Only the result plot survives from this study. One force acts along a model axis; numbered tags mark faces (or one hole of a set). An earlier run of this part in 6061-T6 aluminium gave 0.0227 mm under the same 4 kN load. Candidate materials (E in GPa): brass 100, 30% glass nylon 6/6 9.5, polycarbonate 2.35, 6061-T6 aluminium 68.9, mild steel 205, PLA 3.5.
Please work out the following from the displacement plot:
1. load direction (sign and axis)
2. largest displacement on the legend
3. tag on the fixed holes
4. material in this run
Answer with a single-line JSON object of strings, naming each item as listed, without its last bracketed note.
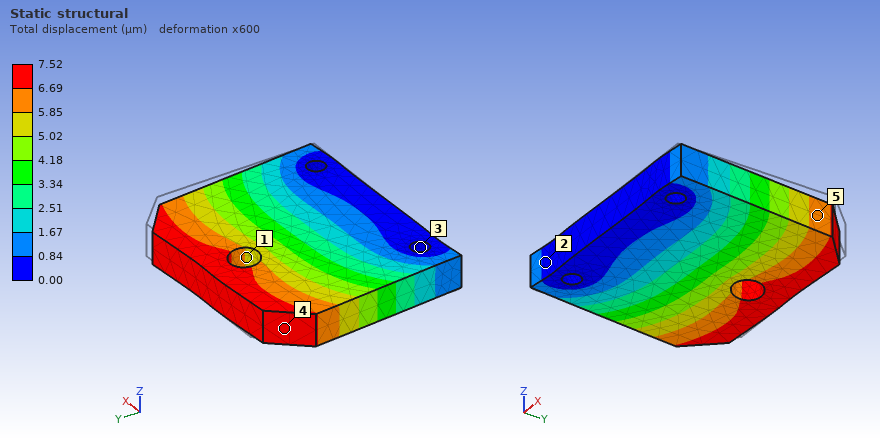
{"load direction": "-X", "largest displacement on the legend": "7.52 µm", "tag on the fixed holes": "3", "material in this run": "mild steel"}
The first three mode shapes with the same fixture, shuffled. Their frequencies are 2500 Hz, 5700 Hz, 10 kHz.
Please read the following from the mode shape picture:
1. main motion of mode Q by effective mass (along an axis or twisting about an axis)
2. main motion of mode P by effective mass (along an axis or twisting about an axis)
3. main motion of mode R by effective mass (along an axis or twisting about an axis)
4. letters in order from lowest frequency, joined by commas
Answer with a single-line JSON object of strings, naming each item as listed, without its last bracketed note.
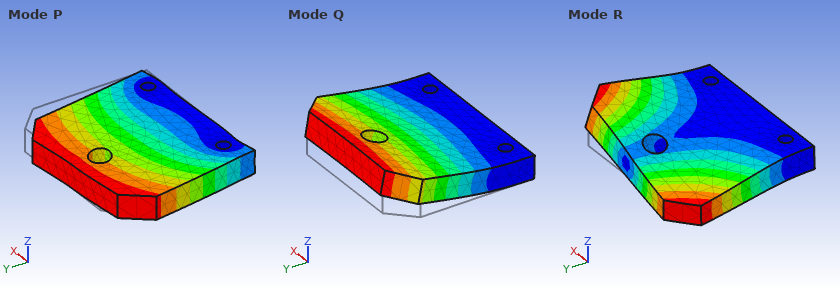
{"main motion of mode Q by effective mass": "along Z", "main motion of mode P by effective mass": "along X", "main motion of mode R by effective mass": "twisting about Y", "letters in order from lowest frequency, joined by commas": "Q, R, P"}
